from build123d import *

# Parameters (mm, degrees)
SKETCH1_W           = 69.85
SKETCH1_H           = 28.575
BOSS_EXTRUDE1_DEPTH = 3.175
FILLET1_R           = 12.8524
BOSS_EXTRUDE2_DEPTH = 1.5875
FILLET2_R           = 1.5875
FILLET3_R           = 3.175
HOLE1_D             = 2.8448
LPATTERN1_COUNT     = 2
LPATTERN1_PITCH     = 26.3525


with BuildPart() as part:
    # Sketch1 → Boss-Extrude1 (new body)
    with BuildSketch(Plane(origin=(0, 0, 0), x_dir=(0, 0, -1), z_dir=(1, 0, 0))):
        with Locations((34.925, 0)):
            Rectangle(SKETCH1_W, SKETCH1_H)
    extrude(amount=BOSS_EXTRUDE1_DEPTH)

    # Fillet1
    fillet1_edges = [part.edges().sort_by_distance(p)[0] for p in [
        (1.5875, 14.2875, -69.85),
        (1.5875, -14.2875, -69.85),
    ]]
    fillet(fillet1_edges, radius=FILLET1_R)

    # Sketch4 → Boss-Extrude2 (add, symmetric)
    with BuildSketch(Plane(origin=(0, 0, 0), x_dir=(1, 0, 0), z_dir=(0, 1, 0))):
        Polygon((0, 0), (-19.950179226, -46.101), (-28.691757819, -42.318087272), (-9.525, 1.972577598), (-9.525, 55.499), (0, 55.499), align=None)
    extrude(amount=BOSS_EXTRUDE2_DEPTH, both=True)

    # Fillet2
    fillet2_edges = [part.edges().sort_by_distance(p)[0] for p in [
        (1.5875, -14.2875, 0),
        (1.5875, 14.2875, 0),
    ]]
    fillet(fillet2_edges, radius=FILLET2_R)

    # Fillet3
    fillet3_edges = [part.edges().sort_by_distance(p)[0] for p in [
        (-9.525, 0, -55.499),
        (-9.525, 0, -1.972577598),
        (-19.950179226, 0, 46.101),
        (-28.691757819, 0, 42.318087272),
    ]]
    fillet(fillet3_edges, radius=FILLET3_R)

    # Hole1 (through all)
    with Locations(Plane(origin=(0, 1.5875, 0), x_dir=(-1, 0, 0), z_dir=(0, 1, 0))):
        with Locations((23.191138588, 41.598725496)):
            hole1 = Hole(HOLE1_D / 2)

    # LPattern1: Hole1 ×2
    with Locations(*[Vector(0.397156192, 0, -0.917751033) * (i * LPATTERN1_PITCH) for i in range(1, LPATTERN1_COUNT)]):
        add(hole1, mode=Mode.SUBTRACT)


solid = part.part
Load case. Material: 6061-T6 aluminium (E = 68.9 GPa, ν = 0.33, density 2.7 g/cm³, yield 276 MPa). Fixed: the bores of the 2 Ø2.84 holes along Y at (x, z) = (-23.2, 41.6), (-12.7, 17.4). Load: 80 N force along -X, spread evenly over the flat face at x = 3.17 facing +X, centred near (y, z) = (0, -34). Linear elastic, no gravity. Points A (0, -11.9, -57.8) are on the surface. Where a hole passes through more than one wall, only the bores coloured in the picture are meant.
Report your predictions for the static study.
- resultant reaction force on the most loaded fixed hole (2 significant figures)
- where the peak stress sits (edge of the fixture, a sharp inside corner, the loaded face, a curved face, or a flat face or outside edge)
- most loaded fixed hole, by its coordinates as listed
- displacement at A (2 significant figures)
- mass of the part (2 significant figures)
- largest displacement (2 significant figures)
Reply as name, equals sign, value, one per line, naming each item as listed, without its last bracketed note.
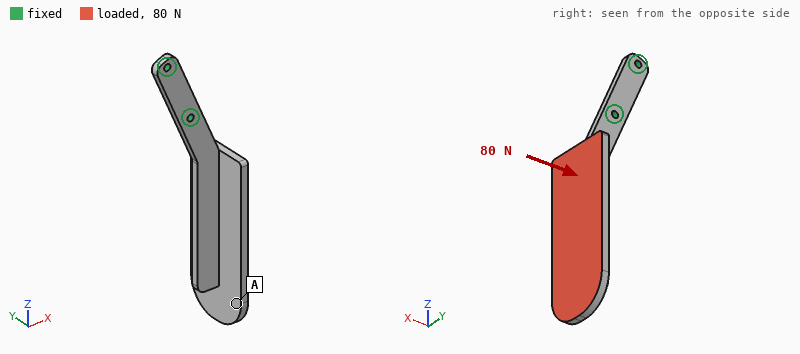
resultant reaction force on the most loaded fixed hole = 150 N
where the peak stress sits = edge of the fixture
most loaded fixed hole, by its coordinates as listed = (-12.7, 17.4)
displacement at A = 0.41 mm
mass of the part = 25 g
largest displacement = 0.49 mm
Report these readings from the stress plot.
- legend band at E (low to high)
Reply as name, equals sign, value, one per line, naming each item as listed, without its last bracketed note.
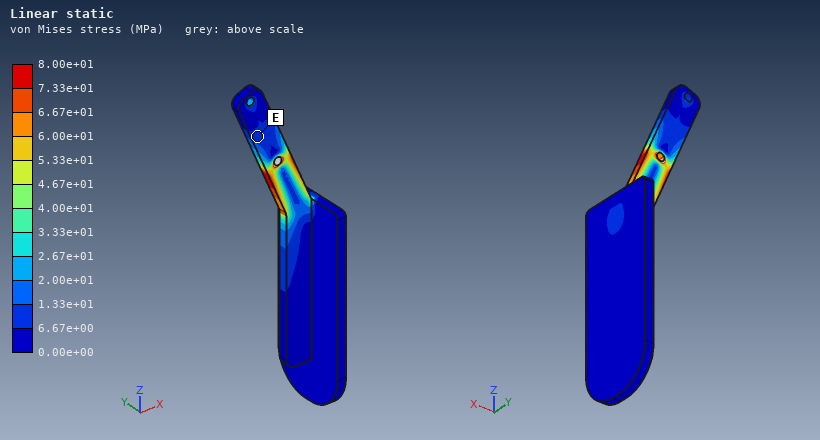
legend band at E = 6.67e+00 to 1.33e+01 MPa
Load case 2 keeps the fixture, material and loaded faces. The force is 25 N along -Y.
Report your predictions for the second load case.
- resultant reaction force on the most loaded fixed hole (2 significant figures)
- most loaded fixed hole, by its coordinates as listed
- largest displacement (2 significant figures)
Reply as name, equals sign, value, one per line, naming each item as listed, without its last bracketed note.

resultant reaction force on the most loaded fixed hole = 28 N
most loaded fixed hole, by its coordinates as listed = (-12.7, 17.4)
largest displacement = 1.1 mm
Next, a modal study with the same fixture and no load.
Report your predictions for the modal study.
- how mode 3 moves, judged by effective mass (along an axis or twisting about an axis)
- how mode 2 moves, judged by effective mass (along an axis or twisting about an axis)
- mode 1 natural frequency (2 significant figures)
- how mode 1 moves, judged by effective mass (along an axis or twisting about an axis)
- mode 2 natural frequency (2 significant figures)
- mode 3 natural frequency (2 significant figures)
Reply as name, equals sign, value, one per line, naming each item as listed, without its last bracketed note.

how mode 3 moves, judged by effective mass = twisting about Z
how mode 2 moves, judged by effective mass = along X
mode 1 natural frequency = 210 Hz
how mode 1 moves, judged by effective mass = along Y
mode 2 natural frequency = 560 Hz
mode 3 natural frequency = 1200 Hz
